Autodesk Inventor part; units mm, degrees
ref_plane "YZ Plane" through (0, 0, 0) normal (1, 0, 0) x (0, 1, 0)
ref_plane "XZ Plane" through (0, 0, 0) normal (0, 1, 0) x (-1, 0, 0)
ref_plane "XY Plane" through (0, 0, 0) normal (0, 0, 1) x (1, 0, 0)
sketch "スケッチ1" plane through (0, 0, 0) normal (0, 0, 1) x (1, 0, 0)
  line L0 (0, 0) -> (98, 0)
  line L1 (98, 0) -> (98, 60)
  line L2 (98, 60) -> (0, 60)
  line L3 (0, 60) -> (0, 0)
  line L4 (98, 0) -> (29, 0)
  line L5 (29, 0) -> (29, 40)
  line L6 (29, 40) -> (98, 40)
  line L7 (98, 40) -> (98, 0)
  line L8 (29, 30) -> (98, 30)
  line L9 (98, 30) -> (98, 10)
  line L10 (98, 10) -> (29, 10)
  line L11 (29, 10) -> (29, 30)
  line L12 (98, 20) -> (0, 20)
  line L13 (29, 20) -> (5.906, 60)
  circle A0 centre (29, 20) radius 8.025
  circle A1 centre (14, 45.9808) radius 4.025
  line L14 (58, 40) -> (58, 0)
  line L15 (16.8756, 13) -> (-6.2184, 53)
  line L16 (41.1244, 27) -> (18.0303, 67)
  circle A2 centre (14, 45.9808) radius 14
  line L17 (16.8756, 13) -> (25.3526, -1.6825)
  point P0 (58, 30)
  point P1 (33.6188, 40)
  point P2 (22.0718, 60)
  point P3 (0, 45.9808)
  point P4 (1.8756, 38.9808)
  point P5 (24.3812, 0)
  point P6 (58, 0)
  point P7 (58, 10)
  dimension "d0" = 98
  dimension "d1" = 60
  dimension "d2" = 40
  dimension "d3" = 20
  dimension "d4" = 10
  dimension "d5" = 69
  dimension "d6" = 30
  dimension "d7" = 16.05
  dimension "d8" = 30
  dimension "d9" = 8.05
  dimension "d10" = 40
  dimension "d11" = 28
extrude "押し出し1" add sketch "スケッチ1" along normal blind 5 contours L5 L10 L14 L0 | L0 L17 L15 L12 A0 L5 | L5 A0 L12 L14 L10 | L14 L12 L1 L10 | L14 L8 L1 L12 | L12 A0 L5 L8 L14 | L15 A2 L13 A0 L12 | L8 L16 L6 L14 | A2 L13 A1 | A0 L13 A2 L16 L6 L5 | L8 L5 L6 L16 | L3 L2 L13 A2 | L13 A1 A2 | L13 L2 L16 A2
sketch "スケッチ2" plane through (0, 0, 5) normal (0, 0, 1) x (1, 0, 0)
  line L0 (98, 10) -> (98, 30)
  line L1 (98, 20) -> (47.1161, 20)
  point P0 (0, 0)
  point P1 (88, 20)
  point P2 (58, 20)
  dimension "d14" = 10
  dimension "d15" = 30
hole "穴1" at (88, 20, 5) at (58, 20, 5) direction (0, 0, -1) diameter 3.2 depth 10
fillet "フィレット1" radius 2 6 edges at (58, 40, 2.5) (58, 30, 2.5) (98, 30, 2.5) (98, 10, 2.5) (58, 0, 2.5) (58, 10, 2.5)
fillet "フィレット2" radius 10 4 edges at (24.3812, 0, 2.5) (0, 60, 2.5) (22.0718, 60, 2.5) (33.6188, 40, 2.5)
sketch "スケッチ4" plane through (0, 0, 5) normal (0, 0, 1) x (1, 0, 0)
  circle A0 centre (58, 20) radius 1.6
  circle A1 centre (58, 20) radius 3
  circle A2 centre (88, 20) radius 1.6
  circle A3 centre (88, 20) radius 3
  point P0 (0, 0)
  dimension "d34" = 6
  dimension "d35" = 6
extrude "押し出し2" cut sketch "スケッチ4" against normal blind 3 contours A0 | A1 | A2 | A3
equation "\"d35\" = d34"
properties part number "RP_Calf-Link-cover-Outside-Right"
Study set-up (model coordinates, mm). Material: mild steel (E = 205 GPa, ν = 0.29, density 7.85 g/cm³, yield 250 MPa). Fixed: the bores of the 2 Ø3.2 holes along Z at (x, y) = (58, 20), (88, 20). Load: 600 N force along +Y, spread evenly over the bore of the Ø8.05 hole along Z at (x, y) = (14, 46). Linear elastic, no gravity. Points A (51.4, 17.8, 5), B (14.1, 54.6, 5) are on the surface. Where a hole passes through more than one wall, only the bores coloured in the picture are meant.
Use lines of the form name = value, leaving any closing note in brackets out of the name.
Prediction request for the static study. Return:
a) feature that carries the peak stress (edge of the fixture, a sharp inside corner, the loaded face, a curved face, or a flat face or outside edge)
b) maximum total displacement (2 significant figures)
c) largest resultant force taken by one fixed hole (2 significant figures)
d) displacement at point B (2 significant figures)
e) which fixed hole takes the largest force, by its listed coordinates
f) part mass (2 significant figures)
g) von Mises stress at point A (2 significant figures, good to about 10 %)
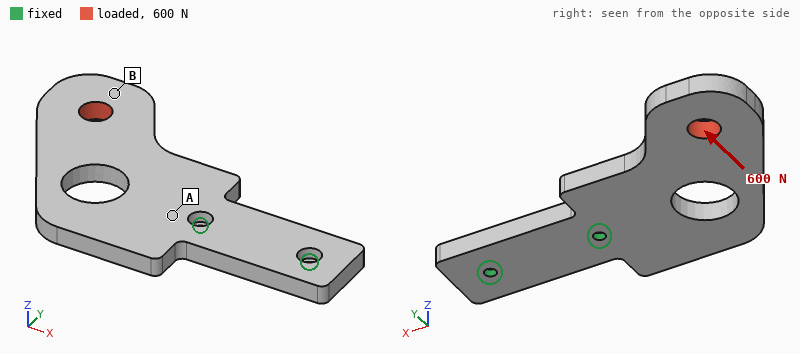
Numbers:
feature that carries the peak stress = edge of the fixture
maximum total displacement = 64 µm
largest resultant force taken by one fixed hole = 1.4 kN
displacement at point B = 54 µm
which fixed hole takes the largest force, by its listed coordinates = (58, 20)
part mass = 110 g
von Mises stress at point A = 36 MPa
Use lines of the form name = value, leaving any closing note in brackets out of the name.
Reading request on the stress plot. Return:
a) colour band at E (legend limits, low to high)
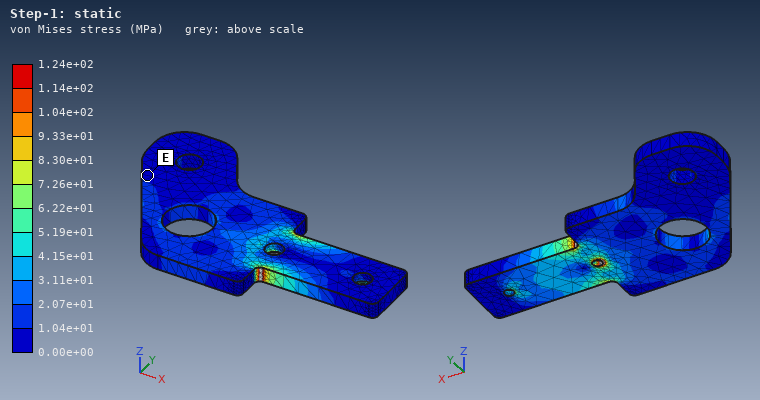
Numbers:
colour band at E = 0.00e+00 to 1.04e+01 MPa
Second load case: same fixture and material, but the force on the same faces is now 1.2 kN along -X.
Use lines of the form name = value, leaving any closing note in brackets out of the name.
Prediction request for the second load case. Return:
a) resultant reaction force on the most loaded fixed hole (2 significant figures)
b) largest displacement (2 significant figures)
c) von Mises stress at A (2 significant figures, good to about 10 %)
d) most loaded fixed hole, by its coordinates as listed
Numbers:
resultant reaction force on the most loaded fixed hole = 1.3 kN
largest displacement = 72 µm
von Mises stress at A = 26 MPa
most loaded fixed hole, by its coordinates as listed = (58, 20)
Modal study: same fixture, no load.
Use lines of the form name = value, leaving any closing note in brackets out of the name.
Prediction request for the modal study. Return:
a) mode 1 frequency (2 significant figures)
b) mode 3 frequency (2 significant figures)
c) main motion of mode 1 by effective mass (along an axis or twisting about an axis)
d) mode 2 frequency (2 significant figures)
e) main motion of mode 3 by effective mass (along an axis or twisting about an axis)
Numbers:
mode 1 frequency = 810 Hz
mode 3 frequency = 2700 Hz
main motion of mode 1 by effective mass = along Z
mode 2 frequency = 2000 Hz
main motion of mode 3 by effective mass = along Y
